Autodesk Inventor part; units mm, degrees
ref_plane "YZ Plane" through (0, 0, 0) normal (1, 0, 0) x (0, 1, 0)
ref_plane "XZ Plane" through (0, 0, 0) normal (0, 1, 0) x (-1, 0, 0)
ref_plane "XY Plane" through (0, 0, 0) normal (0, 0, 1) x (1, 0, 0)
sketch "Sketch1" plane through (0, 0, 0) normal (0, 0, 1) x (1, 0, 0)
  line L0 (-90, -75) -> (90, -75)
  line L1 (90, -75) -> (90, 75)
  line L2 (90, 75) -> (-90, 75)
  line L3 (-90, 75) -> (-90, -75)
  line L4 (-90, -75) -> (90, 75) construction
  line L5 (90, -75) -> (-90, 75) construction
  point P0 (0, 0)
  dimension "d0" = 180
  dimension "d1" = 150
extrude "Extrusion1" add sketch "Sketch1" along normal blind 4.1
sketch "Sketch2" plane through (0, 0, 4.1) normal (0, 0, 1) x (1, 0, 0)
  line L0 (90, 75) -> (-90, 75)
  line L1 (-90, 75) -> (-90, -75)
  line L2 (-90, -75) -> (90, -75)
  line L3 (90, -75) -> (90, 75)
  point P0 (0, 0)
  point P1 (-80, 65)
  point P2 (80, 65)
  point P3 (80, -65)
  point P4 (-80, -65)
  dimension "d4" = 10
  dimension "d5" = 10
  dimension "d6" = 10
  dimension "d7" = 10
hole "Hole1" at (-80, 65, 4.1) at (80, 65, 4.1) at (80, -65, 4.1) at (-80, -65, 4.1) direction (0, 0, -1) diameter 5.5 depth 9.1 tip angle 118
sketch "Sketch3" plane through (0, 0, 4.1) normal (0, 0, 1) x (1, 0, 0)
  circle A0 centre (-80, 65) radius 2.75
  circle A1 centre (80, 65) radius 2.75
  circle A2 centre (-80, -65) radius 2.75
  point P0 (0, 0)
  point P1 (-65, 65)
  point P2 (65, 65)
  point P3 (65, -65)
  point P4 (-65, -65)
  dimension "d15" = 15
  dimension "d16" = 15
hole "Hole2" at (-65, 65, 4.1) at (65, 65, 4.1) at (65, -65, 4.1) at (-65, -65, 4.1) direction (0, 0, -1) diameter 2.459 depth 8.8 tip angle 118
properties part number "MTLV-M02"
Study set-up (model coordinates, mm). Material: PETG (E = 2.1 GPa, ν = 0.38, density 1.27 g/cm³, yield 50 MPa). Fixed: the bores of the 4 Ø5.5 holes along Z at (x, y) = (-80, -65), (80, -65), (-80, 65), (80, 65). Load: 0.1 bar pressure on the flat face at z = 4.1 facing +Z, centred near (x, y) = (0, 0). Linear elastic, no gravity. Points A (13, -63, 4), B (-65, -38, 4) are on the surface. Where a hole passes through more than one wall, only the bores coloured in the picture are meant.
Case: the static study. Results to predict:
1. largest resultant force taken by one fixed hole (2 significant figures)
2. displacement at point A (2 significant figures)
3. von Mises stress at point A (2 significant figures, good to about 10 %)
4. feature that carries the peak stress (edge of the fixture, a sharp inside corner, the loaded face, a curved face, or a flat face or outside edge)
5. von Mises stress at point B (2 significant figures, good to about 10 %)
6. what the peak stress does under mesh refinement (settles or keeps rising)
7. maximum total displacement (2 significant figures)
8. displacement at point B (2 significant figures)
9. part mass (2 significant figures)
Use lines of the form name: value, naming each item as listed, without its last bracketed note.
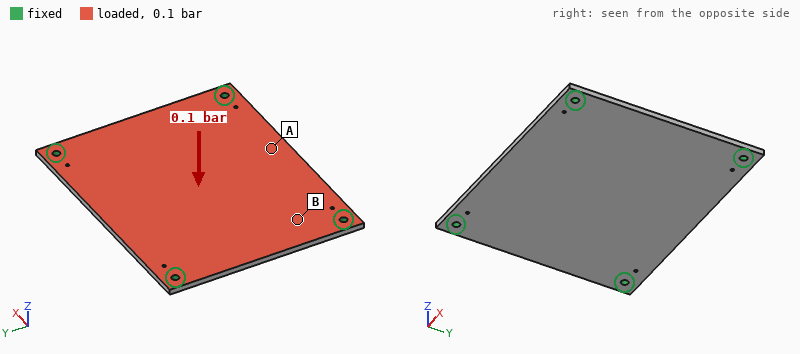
largest resultant force taken by one fixed hole: 67 N
displacement at point A: 2.1 mm
von Mises stress at point A: 4.8 MPa
feature that carries the peak stress: edge of the fixture
von Mises stress at point B: 1.8 MPa
what the peak stress does under mesh refinement: keeps rising
maximum total displacement: 2.8 mm
displacement at point B: 0.88 mm
part mass: 140 g
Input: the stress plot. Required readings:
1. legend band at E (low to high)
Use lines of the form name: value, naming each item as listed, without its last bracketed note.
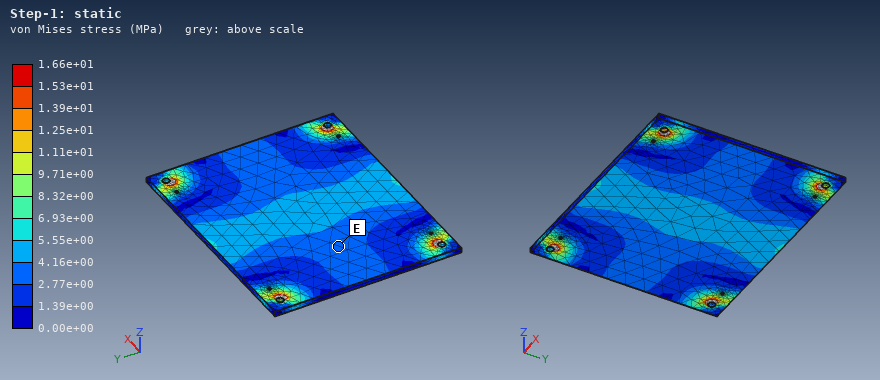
legend band at E: 2.77e+00 to 4.16e+00 MPa
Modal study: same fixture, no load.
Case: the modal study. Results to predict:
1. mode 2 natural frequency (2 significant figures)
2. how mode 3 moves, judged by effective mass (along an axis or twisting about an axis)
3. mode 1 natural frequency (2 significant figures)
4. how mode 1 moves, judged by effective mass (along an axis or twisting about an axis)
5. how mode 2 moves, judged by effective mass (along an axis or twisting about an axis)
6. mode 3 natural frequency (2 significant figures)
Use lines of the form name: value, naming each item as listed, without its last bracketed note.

mode 2 natural frequency: 250 Hz
how mode 3 moves, judged by effective mass: twisting about Y
mode 1 natural frequency: 160 Hz
how mode 1 moves, judged by effective mass: along Z
how mode 2 moves, judged by effective mass: twisting about X
mode 3 natural frequency: 320 Hz
